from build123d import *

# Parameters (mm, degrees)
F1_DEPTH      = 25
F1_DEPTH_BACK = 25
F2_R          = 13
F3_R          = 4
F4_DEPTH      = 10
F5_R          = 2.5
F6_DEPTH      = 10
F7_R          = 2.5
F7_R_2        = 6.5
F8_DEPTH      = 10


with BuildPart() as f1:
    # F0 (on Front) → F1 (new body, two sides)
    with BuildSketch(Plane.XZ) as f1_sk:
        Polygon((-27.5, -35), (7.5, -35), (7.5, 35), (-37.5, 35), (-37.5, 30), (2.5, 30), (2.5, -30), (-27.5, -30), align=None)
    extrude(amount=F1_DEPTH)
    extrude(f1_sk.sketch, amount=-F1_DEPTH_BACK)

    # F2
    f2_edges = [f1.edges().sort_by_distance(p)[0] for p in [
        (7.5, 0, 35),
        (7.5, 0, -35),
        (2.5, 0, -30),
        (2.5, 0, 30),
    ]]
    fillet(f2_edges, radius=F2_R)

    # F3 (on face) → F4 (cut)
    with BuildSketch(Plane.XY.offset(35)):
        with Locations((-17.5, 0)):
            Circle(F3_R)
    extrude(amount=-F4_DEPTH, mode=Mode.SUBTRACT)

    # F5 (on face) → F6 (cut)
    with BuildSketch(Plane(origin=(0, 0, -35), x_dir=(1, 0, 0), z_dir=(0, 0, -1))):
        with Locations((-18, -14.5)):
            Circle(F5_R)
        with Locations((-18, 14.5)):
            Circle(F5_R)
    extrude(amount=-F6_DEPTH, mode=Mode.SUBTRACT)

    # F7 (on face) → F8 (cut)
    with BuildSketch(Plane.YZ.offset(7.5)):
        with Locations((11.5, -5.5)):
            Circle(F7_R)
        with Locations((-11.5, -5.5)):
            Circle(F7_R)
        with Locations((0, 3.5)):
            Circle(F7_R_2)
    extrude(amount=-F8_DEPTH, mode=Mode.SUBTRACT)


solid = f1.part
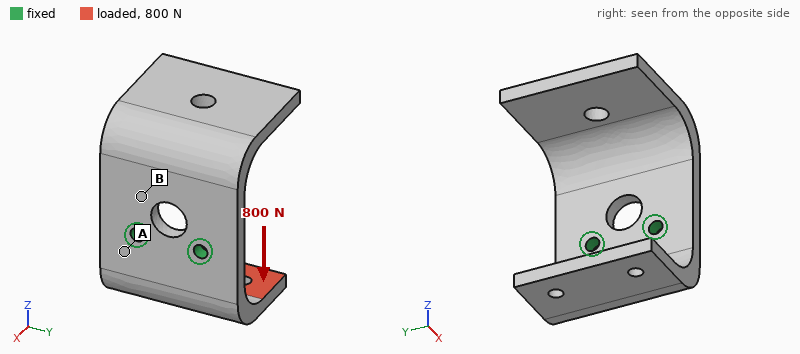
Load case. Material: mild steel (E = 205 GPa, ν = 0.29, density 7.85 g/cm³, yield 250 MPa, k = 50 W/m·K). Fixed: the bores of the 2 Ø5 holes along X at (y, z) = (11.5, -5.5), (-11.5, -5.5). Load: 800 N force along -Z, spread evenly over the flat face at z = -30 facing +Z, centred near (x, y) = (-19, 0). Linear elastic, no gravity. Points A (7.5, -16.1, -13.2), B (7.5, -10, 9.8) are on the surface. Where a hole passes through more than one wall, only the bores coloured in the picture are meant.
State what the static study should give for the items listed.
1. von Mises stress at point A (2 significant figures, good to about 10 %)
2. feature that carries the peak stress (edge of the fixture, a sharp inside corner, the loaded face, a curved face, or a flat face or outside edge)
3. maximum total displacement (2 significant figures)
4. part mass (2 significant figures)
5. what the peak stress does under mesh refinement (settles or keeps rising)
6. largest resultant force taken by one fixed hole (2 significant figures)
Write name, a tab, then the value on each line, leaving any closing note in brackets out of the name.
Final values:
von Mises stress at point A	82 MPa
feature that carries the peak stress	edge of the fixture
maximum total displacement	0.15 mm
part mass	260 g
what the peak stress does under mesh refinement	keeps rising
largest resultant force taken by one fixed hole	420 N
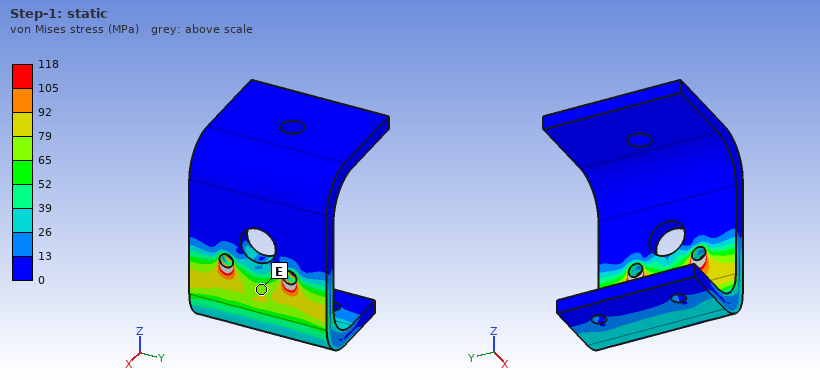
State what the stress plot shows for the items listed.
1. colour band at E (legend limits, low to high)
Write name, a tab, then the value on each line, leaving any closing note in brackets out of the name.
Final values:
colour band at E	65 to 79 MPa
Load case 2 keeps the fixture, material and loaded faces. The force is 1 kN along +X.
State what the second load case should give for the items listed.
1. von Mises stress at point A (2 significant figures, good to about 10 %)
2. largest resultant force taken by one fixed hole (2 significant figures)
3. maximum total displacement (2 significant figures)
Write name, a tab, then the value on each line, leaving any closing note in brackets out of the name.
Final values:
von Mises stress at point A	74 MPa
largest resultant force taken by one fixed hole	500 N
maximum total displacement	98 µm
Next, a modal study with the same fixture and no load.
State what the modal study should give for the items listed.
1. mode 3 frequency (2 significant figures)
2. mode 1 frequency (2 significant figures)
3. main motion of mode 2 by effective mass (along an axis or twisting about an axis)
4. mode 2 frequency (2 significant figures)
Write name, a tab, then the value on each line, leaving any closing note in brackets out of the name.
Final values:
mode 3 frequency	1800 Hz
mode 1 frequency	850 Hz
main motion of mode 2 by effective mass	along Y
mode 2 frequency	1700 Hz
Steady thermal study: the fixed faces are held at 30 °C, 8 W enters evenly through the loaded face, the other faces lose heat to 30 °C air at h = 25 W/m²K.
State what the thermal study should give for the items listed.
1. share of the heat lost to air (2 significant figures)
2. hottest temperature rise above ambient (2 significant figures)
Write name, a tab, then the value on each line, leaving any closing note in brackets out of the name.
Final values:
share of the heat lost to air	23 %
hottest temperature rise above ambient	24 K
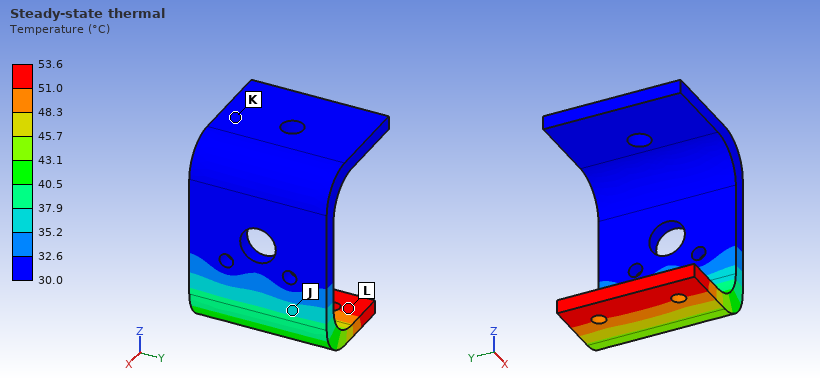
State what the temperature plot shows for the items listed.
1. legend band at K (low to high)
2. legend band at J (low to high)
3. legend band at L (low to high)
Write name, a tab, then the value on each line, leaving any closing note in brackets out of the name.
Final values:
legend band at K	30.0 to 32.6 °C
legend band at J	35.2 to 37.9 °C
legend band at L	51.0 to 53.6 °C
